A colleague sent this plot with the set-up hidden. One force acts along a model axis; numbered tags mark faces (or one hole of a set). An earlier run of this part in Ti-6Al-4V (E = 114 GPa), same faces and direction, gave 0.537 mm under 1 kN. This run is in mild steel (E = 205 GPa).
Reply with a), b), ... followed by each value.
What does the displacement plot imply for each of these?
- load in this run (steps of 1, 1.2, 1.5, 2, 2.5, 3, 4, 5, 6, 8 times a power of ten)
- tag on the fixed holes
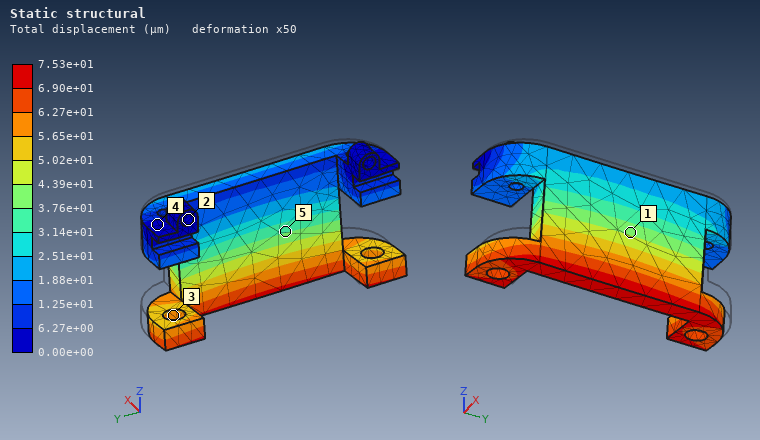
a) 250 N
b) 2
